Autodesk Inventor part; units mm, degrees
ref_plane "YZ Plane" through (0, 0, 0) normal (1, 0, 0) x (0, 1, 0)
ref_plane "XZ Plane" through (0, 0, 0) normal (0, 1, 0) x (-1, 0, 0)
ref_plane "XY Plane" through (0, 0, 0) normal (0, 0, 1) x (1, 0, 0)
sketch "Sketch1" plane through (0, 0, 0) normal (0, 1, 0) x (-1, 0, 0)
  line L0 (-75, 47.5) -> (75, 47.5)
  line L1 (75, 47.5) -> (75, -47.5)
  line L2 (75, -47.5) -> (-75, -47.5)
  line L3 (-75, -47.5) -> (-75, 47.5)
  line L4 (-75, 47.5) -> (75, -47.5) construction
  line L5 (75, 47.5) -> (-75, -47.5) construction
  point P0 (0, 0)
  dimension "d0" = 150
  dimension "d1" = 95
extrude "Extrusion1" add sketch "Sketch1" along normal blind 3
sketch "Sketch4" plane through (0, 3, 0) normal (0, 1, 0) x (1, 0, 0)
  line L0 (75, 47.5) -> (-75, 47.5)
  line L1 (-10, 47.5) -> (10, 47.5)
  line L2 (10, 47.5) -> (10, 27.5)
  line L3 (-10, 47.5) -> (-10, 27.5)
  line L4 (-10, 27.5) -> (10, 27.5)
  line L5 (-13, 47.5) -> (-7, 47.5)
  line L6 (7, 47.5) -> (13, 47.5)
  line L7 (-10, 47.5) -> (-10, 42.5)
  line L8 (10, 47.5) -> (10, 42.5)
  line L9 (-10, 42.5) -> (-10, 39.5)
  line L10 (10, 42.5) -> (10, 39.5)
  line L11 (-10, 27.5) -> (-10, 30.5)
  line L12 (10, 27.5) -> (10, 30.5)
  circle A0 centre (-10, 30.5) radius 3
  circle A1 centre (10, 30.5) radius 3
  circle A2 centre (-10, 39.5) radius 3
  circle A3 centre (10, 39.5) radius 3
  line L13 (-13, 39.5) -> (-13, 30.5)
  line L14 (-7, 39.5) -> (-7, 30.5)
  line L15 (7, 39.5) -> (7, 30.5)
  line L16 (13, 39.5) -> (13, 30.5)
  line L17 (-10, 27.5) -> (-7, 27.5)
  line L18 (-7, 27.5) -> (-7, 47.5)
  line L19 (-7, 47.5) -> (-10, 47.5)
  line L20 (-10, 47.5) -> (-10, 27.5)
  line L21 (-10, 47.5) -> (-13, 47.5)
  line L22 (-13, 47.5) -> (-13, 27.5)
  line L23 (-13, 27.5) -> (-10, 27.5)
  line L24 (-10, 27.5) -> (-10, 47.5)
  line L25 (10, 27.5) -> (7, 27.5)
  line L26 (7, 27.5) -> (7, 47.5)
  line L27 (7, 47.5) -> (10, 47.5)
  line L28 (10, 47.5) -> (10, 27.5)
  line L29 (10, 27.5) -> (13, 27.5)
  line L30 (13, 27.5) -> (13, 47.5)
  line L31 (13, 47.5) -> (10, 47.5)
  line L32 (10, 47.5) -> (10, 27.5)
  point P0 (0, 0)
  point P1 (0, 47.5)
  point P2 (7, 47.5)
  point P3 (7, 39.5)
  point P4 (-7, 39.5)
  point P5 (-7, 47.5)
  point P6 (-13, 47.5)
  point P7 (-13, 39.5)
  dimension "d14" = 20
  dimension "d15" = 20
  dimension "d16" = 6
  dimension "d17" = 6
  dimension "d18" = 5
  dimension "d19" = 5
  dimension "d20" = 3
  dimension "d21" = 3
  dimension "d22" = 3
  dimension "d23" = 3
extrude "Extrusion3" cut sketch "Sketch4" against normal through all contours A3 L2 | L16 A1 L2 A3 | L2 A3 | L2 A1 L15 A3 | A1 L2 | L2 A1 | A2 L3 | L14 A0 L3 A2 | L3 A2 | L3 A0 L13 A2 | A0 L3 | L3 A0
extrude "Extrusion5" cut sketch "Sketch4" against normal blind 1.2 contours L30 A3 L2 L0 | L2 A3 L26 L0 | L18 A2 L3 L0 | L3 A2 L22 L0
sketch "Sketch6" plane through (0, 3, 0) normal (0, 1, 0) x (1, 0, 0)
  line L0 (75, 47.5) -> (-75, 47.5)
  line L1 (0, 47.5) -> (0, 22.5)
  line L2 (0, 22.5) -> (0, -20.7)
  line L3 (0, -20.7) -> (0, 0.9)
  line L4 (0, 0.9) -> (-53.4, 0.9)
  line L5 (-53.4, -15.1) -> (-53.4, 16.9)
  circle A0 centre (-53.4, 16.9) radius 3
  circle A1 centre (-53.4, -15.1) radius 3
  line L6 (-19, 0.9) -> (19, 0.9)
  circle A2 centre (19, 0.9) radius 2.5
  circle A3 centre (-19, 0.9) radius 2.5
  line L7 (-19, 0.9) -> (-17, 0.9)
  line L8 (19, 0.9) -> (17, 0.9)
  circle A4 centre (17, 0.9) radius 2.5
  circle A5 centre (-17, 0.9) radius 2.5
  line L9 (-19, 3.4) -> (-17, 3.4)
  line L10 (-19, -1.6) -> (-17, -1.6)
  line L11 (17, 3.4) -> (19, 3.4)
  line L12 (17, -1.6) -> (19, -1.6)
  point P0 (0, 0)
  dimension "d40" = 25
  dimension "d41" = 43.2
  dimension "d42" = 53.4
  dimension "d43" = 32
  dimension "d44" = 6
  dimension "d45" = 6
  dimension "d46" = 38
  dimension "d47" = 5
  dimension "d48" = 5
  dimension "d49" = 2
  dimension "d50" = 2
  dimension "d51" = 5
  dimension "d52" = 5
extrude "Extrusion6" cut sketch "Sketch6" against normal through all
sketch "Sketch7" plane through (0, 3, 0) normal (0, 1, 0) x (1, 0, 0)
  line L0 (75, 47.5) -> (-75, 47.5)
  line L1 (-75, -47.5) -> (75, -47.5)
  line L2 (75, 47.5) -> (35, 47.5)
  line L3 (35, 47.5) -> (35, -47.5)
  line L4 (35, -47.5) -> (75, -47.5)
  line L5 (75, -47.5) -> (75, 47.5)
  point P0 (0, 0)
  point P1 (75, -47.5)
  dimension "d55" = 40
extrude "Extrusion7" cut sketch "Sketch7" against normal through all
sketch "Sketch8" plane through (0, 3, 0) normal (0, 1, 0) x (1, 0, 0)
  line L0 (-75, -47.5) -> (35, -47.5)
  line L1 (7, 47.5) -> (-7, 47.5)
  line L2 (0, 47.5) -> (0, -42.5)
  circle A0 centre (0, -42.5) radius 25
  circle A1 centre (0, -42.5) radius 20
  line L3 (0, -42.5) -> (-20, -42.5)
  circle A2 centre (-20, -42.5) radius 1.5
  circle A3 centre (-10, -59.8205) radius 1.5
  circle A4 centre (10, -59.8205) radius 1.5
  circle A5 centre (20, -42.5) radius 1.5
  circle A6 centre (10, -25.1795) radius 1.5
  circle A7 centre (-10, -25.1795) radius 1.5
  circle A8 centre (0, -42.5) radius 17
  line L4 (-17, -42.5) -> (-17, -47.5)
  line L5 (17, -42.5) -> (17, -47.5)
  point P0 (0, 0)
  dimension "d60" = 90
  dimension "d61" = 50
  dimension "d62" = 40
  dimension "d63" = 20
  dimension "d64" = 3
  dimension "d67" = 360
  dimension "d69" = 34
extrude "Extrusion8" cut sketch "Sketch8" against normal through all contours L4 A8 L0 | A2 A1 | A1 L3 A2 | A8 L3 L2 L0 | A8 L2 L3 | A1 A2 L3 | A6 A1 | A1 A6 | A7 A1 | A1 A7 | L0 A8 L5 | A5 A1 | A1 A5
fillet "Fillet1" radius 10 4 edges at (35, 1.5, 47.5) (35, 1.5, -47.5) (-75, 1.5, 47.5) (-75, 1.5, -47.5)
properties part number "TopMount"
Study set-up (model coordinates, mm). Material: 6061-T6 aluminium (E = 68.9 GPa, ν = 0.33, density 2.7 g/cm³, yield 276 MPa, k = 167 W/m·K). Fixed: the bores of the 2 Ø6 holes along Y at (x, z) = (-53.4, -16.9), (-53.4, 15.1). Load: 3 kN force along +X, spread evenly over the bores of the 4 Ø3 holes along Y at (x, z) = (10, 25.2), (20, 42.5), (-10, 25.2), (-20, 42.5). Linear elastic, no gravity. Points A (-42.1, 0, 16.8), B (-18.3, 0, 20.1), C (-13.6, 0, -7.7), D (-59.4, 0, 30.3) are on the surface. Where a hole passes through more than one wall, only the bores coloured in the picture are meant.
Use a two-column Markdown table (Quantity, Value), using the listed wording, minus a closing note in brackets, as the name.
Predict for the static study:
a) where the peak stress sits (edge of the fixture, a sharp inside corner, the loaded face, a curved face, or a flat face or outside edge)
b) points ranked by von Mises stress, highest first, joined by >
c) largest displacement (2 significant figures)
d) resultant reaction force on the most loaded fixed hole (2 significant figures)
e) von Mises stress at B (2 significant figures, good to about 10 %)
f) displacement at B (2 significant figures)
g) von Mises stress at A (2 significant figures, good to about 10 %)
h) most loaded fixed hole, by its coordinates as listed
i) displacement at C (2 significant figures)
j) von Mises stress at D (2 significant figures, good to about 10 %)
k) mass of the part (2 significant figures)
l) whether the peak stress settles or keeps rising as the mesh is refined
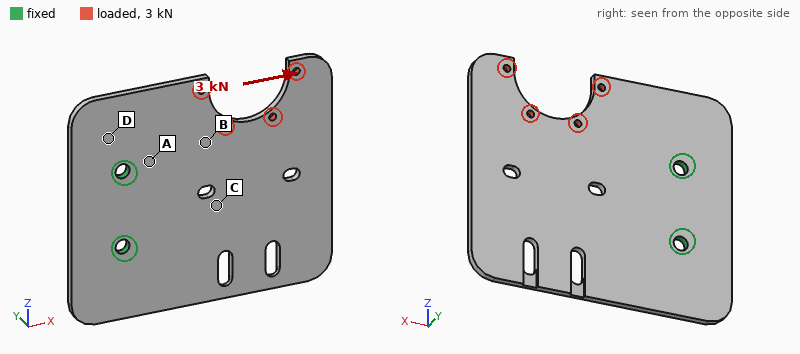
| Quantity | Value |
|---|---|
| where the peak stress sits | edge of the fixture |
| points ranked by von Mises stress, highest first, joined by > | A > B > D > C |
| largest displacement | 0.15 mm |
| resultant reaction force on the most loaded fixed hole | 4.4 kN |
| von Mises stress at B | 42 MPa |
| displacement at B | 0.037 mm |
| von Mises stress at A | 56 MPa |
| most loaded fixed hole, by its coordinates as listed | (-53.4, 15.1) |
| displacement at C | 0.027 mm |
| von Mises stress at D | 19 MPa |
| mass of the part | 76 g |
| whether the peak stress settles or keeps rising as the mesh is refined | keeps rising |
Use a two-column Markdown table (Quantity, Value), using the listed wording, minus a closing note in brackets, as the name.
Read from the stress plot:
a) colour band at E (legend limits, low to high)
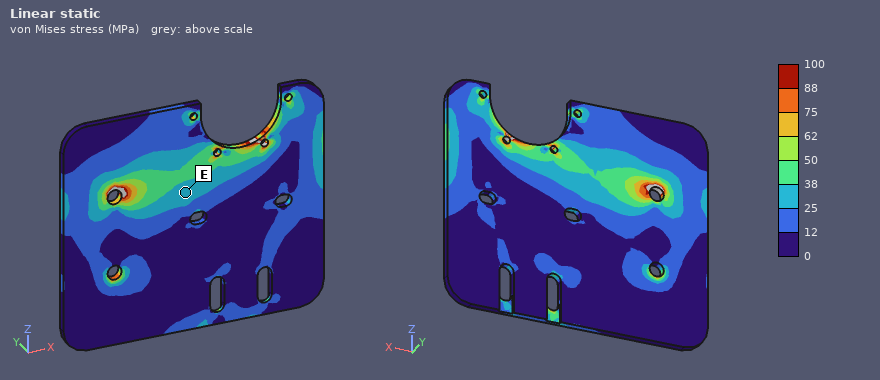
| Quantity | Value |
|---|---|
| colour band at E | 25 to 38 MPa |
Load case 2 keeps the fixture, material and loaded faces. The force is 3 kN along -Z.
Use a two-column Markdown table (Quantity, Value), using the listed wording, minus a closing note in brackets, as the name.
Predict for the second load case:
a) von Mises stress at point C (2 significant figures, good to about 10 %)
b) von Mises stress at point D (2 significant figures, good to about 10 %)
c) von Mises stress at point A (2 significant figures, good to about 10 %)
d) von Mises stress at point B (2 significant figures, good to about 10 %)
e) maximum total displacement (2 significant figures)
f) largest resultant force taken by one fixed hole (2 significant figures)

| Quantity | Value |
|---|---|
| von Mises stress at point C | 25 MPa |
| von Mises stress at point D | 22 MPa |
| von Mises stress at point A | 53 MPa |
| von Mises stress at point B | 33 MPa |
| maximum total displacement | 0.15 mm |
| largest resultant force taken by one fixed hole | 4.7 kN |
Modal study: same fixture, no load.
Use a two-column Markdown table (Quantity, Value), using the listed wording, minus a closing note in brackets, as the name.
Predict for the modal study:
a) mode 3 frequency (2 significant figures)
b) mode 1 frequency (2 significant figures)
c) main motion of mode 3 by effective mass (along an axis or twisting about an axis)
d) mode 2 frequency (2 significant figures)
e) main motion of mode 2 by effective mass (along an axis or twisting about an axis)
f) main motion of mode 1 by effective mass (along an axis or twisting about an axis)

| Quantity | Value |
|---|---|
| mode 3 frequency | 1700 Hz |
| mode 1 frequency | 310 Hz |
| main motion of mode 3 by effective mass | along Y |
| mode 2 frequency | 690 Hz |
| main motion of mode 2 by effective mass | twisting about X |
| main motion of mode 1 by effective mass | along Y |
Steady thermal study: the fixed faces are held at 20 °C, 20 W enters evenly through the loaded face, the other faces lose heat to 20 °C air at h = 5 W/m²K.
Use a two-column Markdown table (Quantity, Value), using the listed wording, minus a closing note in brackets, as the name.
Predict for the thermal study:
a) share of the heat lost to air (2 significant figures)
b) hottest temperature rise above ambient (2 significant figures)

| Quantity | Value |
|---|---|
| share of the heat lost to air | 7.9 % |
| hottest temperature rise above ambient | 50 K |
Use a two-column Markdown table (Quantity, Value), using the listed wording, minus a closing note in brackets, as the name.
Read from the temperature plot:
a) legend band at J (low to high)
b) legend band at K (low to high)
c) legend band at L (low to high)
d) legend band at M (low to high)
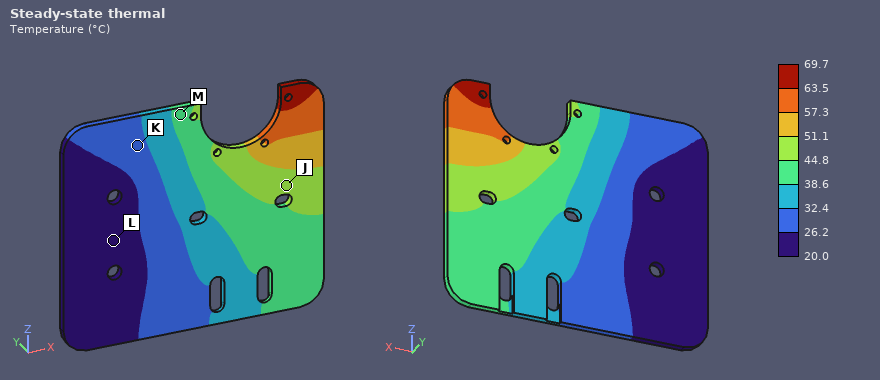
| Quantity | Value |
|---|---|
| legend band at J | 44.8 to 51.1 °C |
| legend band at K | 26.2 to 32.4 °C |
| legend band at L | 20.0 to 26.2 °C |
| legend band at M | 38.6 to 44.8 °C |
